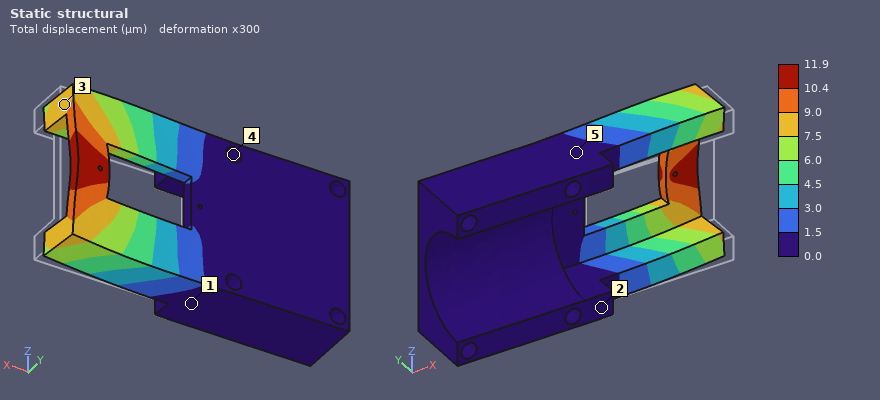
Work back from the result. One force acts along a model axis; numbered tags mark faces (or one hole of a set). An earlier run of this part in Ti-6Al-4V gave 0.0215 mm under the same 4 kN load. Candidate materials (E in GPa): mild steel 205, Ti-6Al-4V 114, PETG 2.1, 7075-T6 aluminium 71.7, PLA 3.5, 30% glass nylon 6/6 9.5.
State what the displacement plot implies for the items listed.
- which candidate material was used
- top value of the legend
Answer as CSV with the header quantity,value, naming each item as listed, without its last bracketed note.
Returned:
quantity,value
which candidate material was used,mild steel
top value of the legend,11.9 µm
